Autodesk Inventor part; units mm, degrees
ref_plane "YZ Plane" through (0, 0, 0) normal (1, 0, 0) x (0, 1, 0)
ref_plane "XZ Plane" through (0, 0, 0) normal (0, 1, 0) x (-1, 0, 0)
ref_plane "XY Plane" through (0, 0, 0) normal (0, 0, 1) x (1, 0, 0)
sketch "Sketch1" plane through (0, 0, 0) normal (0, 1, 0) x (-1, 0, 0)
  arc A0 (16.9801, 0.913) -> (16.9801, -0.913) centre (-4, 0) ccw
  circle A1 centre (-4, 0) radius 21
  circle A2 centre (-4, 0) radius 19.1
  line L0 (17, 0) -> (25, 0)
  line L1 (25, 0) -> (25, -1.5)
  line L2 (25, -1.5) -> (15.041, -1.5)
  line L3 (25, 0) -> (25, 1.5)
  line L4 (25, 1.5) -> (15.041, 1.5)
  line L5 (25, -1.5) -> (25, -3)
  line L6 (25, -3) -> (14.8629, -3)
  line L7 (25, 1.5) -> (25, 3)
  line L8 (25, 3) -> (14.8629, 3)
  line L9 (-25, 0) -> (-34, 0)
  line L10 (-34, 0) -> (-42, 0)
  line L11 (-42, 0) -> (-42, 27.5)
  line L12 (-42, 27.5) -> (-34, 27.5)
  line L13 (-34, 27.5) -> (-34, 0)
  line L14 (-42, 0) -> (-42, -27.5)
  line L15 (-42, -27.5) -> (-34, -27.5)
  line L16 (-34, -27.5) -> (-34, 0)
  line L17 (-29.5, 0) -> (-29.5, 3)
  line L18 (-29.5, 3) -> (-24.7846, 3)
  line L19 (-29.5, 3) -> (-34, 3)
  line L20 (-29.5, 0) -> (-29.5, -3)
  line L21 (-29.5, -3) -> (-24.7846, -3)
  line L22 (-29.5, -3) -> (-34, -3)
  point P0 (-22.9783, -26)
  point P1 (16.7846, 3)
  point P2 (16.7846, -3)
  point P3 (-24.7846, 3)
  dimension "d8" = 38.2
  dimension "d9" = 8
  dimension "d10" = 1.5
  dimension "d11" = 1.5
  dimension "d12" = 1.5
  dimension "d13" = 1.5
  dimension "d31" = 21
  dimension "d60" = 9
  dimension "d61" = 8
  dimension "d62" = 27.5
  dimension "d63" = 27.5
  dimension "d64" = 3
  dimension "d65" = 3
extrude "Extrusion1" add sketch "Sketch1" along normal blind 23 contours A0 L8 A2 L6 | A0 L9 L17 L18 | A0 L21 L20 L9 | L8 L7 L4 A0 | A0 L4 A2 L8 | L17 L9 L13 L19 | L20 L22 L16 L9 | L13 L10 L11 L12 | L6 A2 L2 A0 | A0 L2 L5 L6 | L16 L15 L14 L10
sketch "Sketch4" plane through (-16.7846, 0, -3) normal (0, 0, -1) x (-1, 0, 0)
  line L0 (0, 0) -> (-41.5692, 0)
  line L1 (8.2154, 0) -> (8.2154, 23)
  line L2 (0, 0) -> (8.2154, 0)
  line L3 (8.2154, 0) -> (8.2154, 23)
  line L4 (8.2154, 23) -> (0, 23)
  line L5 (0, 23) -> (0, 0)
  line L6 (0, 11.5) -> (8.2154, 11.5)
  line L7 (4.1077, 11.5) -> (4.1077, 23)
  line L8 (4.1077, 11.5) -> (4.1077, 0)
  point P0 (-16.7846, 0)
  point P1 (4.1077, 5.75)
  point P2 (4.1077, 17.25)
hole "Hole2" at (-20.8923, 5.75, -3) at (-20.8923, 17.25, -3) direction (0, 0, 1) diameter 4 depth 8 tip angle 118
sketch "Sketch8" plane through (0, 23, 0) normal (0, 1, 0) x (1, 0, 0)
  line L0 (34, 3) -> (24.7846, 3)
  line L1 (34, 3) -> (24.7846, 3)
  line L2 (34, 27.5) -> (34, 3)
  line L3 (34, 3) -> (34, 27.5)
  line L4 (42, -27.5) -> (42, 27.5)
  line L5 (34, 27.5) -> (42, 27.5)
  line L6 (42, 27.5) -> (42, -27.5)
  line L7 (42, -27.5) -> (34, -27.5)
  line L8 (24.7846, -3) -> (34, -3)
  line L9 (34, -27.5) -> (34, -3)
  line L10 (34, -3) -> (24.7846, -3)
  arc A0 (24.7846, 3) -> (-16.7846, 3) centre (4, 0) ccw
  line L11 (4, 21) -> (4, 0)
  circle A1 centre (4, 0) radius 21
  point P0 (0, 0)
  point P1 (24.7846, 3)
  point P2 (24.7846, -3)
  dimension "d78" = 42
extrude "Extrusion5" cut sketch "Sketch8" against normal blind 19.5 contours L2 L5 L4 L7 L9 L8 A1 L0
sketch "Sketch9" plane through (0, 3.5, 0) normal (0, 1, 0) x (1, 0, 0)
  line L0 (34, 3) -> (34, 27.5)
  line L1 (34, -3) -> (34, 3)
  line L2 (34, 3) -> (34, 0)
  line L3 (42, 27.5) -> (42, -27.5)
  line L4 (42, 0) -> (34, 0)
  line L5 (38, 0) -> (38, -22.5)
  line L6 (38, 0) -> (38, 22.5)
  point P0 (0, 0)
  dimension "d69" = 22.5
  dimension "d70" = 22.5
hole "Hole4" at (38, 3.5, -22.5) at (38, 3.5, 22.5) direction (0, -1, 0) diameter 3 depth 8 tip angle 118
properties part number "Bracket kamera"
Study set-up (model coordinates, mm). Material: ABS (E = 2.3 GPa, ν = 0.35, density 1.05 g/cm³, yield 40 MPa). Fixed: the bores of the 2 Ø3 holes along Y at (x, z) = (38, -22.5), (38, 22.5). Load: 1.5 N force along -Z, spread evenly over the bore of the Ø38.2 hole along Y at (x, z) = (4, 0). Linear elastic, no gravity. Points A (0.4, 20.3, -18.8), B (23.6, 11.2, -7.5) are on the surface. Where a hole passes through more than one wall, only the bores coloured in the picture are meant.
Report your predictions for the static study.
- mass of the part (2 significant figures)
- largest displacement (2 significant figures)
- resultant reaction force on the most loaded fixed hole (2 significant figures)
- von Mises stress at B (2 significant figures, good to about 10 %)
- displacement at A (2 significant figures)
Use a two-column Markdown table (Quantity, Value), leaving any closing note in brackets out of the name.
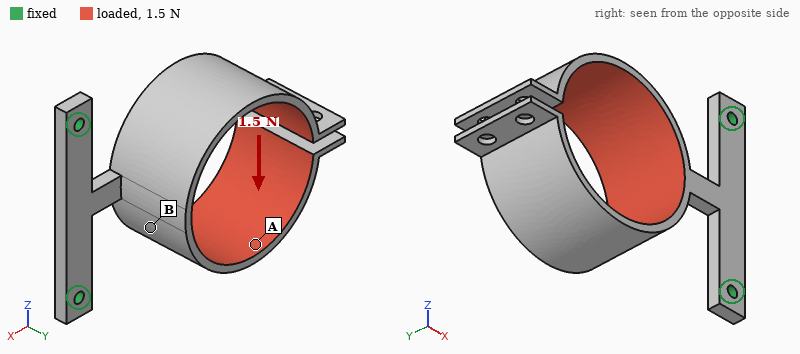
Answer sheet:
| Quantity | Value |
|---|---|
| mass of the part | 7.9 g |
| largest displacement | 0.91 mm |
| resultant reaction force on the most loaded fixed hole | 1.7 N |
| von Mises stress at B | 0.89 MPa |
| displacement at A | 0.50 mm |
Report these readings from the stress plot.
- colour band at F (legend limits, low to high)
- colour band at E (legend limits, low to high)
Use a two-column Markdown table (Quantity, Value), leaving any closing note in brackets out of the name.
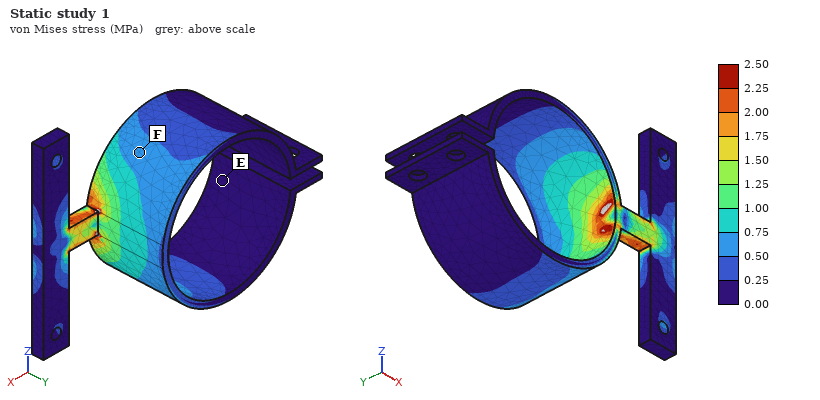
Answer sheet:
| Quantity | Value |
|---|---|
| colour band at F | 0.50 to 0.75 MPa |
| colour band at E | 0.00 to 0.25 MPa |
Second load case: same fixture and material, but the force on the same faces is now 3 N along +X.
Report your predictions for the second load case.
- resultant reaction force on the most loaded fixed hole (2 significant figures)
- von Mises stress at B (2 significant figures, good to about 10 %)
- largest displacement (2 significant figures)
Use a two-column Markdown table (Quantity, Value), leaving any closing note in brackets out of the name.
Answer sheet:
| Quantity | Value |
|---|---|
| resultant reaction force on the most loaded fixed hole | 1.5 N |
| von Mises stress at B | 0.55 MPa |
| largest displacement | 0.87 mm |
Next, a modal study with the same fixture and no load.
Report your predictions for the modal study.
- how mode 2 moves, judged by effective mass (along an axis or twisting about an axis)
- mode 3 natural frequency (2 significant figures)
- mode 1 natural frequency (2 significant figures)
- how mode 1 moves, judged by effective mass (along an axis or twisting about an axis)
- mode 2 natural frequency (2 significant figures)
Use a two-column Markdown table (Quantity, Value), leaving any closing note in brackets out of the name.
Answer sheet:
| Quantity | Value |
|---|---|
| how mode 2 moves, judged by effective mass | along Z |
| mode 3 natural frequency | 130 Hz |
| mode 1 natural frequency | 78 Hz |
| how mode 1 moves, judged by effective mass | along Y |
| mode 2 natural frequency | 94 Hz |
